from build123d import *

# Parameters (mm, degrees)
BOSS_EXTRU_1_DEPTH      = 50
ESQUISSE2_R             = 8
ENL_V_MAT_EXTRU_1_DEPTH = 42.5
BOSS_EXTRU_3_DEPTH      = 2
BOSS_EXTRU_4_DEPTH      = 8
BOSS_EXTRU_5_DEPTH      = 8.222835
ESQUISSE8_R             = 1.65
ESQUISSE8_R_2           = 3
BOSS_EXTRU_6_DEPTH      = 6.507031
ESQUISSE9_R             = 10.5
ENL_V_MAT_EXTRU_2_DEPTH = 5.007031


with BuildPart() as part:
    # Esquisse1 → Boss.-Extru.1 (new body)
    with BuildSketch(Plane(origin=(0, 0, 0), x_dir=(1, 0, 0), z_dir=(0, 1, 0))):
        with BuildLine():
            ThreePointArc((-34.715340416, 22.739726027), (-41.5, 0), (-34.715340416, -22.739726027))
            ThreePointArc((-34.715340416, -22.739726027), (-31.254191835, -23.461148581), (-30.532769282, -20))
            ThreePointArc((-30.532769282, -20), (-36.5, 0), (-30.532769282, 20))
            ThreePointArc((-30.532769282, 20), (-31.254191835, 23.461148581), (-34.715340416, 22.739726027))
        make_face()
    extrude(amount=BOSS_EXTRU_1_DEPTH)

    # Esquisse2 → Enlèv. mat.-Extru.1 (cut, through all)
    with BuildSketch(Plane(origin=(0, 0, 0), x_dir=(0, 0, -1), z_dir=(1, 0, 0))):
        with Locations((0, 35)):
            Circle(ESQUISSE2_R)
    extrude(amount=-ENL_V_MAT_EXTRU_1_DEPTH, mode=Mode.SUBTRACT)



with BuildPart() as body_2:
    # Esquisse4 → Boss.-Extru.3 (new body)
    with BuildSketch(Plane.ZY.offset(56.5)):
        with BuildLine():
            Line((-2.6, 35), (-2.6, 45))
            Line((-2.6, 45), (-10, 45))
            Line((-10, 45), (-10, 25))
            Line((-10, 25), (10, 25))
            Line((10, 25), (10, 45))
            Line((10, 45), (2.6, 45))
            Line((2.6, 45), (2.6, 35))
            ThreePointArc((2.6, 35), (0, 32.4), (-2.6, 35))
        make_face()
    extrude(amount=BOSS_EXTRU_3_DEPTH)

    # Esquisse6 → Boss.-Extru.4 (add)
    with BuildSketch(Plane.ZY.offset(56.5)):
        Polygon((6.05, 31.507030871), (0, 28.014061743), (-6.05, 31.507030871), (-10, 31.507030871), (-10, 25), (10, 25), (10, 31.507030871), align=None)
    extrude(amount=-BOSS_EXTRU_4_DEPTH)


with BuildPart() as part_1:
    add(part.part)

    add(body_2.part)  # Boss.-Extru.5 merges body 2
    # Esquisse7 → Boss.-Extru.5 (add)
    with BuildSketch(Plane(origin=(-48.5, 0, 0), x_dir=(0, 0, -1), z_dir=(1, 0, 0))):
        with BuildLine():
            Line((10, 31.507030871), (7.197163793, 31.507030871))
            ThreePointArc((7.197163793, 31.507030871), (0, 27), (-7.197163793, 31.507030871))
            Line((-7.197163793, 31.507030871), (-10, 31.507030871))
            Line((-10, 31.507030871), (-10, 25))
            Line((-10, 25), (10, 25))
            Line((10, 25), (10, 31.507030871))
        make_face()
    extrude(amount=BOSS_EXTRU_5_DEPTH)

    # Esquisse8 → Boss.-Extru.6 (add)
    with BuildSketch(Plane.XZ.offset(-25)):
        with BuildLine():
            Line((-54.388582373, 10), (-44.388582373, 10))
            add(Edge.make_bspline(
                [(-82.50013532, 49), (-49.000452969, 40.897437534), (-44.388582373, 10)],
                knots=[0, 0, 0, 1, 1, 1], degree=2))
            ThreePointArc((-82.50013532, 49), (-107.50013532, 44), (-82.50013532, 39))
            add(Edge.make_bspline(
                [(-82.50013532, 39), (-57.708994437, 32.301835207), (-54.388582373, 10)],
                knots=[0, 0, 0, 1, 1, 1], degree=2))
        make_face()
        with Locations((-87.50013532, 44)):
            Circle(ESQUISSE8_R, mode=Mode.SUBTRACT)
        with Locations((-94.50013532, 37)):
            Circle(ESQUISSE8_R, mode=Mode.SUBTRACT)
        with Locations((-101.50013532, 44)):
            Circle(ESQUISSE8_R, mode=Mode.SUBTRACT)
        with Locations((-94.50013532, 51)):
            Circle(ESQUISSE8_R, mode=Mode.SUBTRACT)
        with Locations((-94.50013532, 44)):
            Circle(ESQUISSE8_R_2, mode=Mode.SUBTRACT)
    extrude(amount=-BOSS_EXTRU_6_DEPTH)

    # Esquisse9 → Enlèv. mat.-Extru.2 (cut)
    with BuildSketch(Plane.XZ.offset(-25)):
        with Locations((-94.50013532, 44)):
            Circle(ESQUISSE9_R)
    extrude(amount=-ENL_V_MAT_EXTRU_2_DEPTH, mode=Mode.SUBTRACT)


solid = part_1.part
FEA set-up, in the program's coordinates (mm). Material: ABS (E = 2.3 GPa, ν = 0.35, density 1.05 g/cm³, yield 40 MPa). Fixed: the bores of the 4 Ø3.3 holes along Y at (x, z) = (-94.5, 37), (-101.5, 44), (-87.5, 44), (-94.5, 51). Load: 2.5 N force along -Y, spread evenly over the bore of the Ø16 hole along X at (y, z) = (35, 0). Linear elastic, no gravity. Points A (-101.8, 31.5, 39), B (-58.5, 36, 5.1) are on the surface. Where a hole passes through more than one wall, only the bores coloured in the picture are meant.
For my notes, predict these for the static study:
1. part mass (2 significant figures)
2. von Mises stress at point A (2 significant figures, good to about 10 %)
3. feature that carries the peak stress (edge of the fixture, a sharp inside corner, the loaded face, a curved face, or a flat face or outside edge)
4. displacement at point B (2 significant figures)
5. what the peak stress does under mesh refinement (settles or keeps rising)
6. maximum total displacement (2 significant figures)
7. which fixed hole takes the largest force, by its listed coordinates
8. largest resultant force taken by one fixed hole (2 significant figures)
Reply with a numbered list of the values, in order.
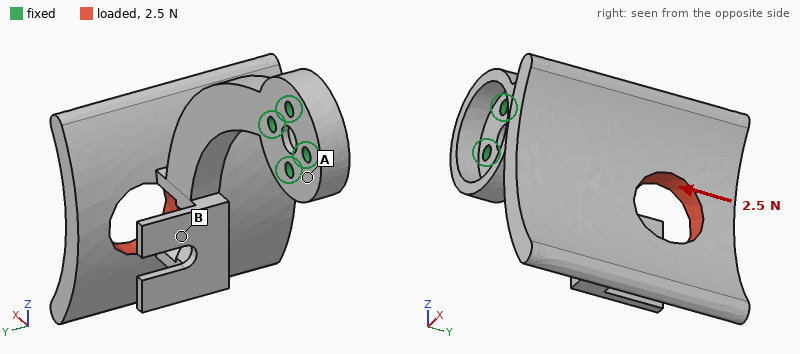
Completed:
1. 19 g
2. 0.66 MPa
3. edge of the fixture
4. 0.59 mm
5. keeps rising
6. 1.4 mm
7. (-87.5, 44)
8. 17 N
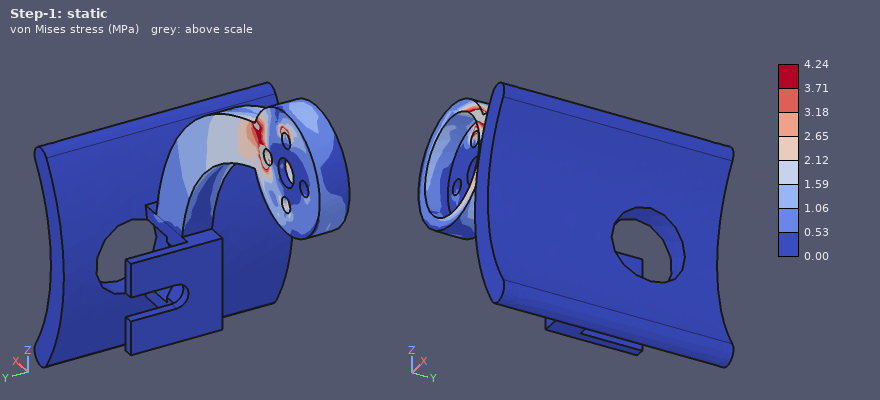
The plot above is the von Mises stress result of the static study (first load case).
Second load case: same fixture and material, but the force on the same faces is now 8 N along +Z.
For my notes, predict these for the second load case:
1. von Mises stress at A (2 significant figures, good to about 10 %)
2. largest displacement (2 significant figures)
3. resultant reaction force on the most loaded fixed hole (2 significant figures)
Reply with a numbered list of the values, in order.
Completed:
1. 0.70 MPa
2. 1.2 mm
3. 23 N
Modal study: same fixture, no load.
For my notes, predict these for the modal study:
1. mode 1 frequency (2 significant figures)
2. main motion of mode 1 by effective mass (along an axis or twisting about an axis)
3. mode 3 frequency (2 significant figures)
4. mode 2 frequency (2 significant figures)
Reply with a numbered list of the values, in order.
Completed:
1. 66 Hz
2. along Y
3. 190 Hz
4. 120 Hz
